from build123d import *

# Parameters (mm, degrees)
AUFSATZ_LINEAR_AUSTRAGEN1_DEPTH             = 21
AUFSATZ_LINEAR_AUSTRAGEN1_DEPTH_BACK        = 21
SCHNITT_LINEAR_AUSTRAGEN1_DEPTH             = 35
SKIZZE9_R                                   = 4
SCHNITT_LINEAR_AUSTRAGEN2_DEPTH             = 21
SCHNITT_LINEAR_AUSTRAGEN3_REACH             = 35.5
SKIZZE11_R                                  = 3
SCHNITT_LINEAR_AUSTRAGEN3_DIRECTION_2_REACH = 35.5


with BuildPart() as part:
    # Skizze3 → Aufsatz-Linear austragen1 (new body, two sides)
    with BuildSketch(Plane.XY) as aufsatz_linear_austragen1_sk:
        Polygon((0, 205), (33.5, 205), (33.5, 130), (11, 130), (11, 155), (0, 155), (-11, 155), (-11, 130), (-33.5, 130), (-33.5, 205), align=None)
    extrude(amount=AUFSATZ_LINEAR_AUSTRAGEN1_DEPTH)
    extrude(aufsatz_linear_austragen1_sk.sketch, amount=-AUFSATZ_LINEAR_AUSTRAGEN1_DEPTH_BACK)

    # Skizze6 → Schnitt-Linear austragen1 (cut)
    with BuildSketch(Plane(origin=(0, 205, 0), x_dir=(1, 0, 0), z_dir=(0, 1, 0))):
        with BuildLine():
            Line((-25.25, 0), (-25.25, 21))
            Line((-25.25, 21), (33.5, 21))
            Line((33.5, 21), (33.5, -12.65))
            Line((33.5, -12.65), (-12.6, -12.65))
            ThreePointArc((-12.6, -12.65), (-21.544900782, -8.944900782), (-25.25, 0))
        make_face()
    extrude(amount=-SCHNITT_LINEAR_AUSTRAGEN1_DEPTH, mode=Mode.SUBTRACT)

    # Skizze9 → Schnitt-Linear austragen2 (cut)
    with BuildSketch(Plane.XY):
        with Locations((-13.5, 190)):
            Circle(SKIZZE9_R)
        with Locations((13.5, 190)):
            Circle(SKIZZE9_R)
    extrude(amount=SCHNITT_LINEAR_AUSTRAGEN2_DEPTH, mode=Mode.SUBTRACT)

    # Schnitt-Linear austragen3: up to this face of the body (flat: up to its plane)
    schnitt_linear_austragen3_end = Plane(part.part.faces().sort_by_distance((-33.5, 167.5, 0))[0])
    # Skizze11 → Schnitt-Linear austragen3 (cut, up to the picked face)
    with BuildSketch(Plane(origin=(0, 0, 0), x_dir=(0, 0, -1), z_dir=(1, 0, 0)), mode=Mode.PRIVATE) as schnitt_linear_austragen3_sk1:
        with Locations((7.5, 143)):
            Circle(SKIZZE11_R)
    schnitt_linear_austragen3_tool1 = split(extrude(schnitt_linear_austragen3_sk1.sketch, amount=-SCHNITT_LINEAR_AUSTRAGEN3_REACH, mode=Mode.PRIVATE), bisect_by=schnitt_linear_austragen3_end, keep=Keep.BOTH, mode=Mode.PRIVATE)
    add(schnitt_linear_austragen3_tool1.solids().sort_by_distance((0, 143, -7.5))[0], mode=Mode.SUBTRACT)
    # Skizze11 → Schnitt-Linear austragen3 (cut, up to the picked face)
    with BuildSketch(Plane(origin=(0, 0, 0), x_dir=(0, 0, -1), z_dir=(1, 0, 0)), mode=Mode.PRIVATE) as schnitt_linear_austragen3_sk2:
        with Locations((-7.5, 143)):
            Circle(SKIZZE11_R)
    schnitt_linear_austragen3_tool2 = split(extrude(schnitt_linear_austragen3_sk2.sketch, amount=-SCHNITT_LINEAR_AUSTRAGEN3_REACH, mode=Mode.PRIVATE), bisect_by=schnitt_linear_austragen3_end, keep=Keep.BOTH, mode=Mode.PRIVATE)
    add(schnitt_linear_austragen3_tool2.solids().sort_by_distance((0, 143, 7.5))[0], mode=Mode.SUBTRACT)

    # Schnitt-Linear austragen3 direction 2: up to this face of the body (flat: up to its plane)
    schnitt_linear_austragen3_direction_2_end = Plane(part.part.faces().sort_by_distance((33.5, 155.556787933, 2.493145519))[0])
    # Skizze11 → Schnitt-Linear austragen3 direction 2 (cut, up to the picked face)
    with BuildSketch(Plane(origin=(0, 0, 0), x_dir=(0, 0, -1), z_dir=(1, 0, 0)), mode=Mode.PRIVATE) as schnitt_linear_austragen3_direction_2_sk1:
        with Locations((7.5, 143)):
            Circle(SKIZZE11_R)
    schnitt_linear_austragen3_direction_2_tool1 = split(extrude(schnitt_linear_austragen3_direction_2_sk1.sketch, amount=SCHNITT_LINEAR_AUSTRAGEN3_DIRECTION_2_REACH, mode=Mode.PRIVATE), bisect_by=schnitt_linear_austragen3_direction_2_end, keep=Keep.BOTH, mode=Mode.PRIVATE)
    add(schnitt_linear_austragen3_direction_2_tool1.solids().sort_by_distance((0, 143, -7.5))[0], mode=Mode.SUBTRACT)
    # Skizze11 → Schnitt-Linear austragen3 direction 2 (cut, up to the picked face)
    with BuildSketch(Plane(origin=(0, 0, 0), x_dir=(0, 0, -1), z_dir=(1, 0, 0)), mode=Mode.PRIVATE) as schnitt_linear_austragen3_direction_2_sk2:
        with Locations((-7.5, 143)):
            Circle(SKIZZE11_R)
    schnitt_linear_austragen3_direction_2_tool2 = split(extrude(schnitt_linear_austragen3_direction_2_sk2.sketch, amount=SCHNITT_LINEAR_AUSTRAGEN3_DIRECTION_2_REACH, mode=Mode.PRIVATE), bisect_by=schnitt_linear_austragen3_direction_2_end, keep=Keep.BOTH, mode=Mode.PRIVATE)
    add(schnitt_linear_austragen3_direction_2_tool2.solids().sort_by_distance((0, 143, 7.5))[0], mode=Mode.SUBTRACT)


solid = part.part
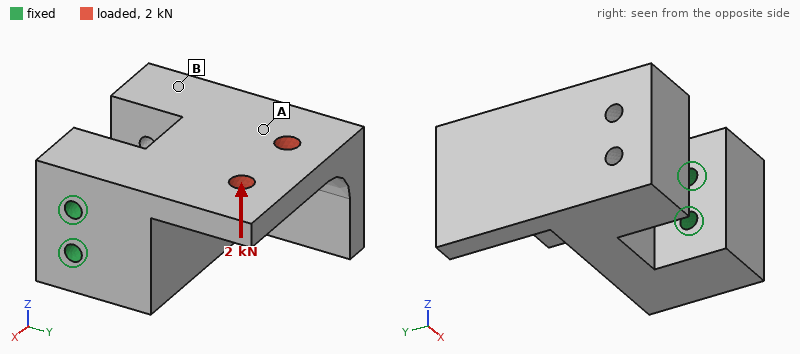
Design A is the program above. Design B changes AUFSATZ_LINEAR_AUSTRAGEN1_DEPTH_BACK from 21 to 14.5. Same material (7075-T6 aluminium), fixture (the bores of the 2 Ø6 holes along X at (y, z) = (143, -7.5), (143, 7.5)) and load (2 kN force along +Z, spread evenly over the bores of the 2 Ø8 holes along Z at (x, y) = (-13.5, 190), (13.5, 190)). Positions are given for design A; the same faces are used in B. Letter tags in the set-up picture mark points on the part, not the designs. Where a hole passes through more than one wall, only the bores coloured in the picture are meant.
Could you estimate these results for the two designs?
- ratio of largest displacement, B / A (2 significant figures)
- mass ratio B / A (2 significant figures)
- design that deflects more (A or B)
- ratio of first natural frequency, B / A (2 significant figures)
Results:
1.1
0.87
B
1.0
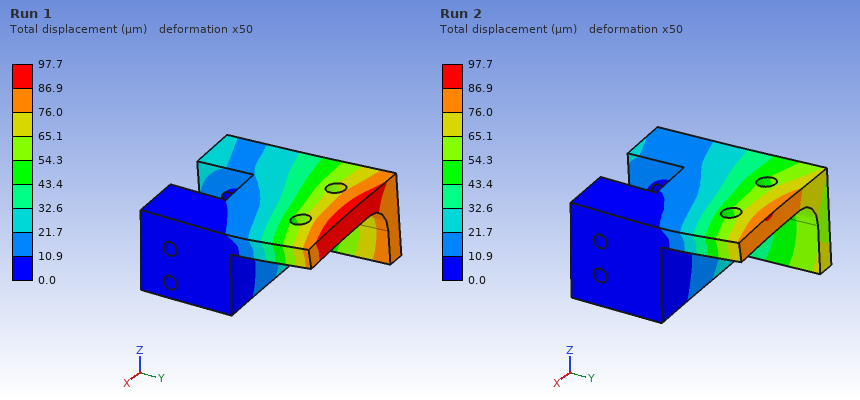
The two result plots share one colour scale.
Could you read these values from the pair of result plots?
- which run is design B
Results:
Run 1
